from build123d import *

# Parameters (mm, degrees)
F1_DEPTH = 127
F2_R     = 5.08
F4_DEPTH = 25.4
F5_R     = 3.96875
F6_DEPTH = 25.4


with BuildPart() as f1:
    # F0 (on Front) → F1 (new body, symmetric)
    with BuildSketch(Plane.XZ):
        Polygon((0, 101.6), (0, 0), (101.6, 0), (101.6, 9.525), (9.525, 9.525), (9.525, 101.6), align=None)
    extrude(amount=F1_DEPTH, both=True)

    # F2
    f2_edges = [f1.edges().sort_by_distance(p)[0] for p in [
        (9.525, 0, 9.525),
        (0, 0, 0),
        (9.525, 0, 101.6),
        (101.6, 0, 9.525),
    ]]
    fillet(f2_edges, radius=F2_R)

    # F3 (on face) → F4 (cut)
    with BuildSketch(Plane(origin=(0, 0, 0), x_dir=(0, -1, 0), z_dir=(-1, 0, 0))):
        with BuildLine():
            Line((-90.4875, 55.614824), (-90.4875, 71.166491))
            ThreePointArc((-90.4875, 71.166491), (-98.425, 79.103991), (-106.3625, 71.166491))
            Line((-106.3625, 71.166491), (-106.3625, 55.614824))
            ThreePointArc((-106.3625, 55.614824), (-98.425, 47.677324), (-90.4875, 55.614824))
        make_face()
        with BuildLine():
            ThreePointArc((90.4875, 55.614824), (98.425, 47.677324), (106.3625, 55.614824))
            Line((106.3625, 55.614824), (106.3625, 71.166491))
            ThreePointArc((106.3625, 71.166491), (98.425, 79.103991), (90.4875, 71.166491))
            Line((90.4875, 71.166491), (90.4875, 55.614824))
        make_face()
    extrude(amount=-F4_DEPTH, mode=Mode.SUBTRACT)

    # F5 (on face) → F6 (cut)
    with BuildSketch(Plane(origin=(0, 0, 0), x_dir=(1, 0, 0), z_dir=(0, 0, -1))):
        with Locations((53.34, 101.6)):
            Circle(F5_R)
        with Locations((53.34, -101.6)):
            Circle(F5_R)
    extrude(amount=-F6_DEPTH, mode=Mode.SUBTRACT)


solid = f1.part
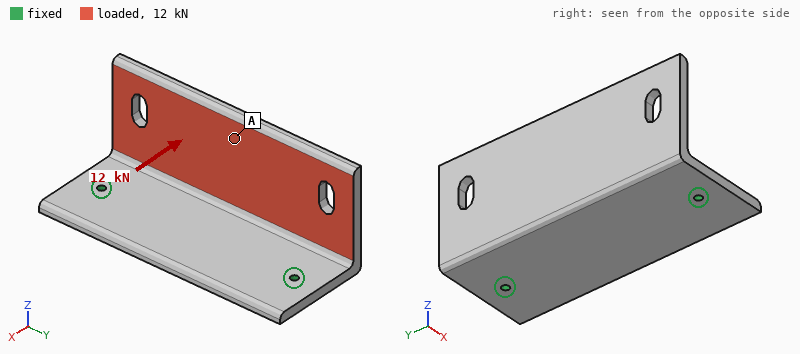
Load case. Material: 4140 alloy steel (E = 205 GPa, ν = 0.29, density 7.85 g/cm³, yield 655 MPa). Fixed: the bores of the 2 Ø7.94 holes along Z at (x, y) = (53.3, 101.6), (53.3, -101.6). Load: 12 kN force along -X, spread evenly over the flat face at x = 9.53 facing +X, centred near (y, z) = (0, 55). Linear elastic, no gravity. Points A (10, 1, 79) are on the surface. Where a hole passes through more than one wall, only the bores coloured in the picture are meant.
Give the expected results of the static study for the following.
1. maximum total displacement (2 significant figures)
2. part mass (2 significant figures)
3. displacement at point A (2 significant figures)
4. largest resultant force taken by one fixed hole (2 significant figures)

1.4 mm
3.6 kg
1.0 mm
6.1 kN
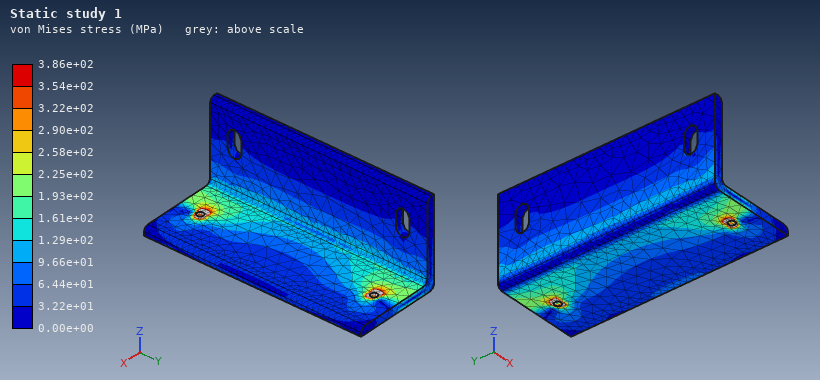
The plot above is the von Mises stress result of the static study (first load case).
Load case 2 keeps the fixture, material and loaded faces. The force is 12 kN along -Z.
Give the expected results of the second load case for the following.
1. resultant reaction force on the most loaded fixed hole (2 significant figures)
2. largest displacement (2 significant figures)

6.1 kN
0.58 mm
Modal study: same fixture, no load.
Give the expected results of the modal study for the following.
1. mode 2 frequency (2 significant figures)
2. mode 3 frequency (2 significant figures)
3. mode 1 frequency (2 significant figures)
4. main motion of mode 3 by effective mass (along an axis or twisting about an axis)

780 Hz
1100 Hz
400 Hz
along Z
